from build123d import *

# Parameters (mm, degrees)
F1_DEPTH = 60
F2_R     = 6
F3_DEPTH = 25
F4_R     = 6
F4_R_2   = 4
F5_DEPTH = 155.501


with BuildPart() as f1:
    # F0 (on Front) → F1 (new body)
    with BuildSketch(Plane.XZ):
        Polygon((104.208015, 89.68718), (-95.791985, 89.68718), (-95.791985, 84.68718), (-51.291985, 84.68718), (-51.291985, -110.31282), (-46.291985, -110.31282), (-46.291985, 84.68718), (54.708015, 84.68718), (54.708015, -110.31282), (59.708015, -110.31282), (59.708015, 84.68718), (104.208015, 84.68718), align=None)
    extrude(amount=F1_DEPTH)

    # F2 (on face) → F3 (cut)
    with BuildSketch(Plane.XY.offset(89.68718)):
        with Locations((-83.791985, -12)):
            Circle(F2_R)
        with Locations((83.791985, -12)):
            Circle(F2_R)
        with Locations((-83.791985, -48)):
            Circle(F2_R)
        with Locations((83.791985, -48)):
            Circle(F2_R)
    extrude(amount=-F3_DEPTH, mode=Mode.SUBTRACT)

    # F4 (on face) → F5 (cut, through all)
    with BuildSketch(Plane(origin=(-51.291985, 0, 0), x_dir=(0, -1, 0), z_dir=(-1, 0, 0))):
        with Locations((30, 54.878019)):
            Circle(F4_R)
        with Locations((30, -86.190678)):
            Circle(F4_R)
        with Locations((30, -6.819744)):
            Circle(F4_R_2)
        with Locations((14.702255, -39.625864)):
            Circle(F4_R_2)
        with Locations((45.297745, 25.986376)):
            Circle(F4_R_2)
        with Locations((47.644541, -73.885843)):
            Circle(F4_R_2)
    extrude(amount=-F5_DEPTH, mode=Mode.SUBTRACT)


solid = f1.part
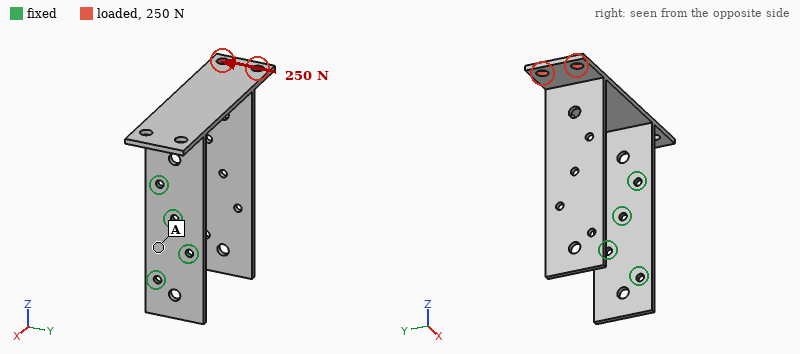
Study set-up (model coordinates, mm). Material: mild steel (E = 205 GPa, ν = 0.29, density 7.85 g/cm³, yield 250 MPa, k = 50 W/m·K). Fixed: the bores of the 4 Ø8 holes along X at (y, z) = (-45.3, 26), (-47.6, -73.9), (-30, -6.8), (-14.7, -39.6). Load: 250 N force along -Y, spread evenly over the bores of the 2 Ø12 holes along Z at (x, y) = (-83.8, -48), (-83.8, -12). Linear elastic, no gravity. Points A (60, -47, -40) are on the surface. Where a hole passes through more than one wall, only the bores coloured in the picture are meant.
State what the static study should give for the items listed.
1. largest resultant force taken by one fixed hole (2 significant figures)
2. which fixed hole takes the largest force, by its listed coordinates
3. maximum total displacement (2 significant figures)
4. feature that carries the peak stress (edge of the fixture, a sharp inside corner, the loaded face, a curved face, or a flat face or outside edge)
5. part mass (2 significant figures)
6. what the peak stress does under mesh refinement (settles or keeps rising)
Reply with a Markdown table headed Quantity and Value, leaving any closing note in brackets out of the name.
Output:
| Quantity | Value |
|---|---|
| largest resultant force taken by one fixed hole | 500 N |
| which fixed hole takes the largest force, by its listed coordinates | (-45.3, 26) |
| maximum total displacement | 1.7 mm |
| feature that carries the peak stress | edge of the fixture |
| part mass | 1.3 kg |
| what the peak stress does under mesh refinement | keeps rising |
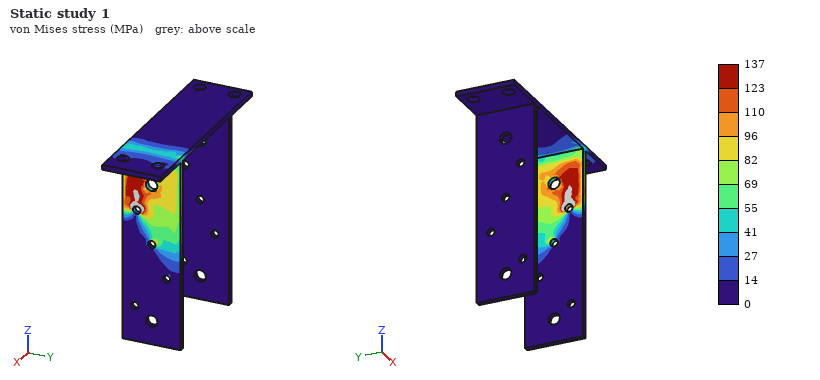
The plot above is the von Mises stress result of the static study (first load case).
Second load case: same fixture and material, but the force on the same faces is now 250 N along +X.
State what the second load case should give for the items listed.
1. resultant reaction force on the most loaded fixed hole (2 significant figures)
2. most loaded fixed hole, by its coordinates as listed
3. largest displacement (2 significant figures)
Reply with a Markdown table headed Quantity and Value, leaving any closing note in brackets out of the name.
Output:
| Quantity | Value |
|---|---|
| resultant reaction force on the most loaded fixed hole | 400 N |
| most loaded fixed hole, by its coordinates as listed | (-45.3, 26) |
| largest displacement | 0.79 mm |
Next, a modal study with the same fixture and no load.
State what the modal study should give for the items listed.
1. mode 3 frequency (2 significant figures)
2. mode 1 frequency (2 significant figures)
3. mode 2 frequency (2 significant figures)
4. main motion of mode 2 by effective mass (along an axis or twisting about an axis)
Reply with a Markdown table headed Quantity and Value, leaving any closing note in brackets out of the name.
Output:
| Quantity | Value |
|---|---|
| mode 3 frequency | 120 Hz |
| mode 1 frequency | 45 Hz |
| mode 2 frequency | 74 Hz |
| main motion of mode 2 by effective mass | along Y |
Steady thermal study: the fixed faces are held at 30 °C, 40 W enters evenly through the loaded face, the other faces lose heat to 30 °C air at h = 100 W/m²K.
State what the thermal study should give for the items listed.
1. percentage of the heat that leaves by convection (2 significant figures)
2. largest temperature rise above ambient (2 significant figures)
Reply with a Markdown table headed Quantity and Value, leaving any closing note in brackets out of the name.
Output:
| Quantity | Value |
|---|---|
| percentage of the heat that leaves by convection | 100 % |
| largest temperature rise above ambient | 75 K |
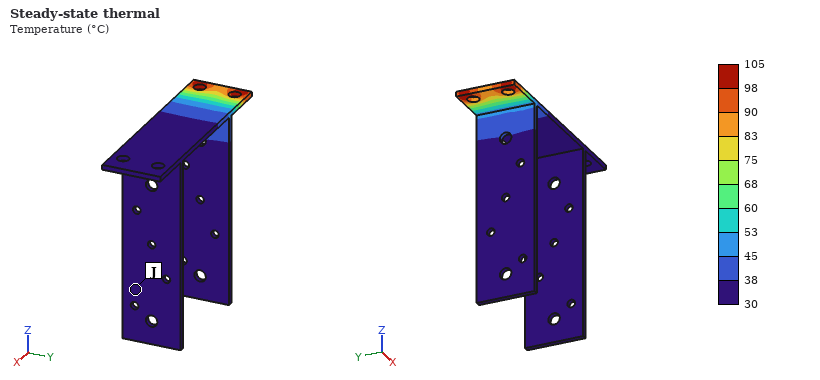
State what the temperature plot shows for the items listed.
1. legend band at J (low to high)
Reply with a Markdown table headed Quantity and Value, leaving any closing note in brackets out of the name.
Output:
| Quantity | Value |
|---|---|
| legend band at J | 30 to 38 °C |
